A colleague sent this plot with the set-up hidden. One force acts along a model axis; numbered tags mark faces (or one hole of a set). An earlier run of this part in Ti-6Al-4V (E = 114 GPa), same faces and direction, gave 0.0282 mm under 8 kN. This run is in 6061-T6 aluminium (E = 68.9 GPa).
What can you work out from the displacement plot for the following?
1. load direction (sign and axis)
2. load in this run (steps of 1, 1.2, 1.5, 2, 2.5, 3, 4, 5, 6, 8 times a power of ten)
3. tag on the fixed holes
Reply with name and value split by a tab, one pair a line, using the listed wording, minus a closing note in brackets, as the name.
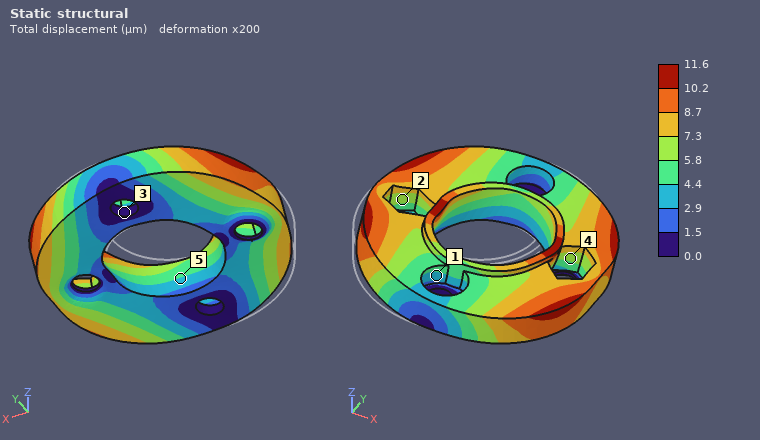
load direction	+X
load in this run	2 kN
tag on the fixed holes	3
